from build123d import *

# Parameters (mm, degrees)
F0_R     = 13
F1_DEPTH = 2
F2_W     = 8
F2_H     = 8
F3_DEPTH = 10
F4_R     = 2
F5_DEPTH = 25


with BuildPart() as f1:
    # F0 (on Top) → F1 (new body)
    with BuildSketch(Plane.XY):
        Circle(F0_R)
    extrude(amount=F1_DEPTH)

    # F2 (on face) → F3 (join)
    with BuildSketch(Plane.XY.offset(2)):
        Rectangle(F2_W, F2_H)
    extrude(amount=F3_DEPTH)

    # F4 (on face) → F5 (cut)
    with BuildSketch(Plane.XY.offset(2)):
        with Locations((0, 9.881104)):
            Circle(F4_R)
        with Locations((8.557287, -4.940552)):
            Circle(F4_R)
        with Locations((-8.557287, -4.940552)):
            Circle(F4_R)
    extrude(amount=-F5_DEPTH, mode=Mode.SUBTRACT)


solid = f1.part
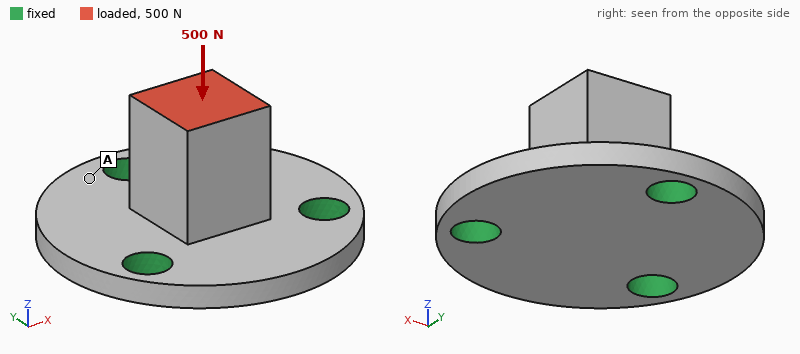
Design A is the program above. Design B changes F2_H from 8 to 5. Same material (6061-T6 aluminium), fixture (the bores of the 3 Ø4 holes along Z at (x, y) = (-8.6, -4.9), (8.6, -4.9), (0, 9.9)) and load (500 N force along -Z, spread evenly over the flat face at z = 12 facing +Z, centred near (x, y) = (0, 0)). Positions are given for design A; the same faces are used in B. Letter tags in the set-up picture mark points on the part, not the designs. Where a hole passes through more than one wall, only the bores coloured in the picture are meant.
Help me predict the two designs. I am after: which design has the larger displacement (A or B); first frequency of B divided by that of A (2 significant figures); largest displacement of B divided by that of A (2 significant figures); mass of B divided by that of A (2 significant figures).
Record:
B
0.91
1.5
0.85
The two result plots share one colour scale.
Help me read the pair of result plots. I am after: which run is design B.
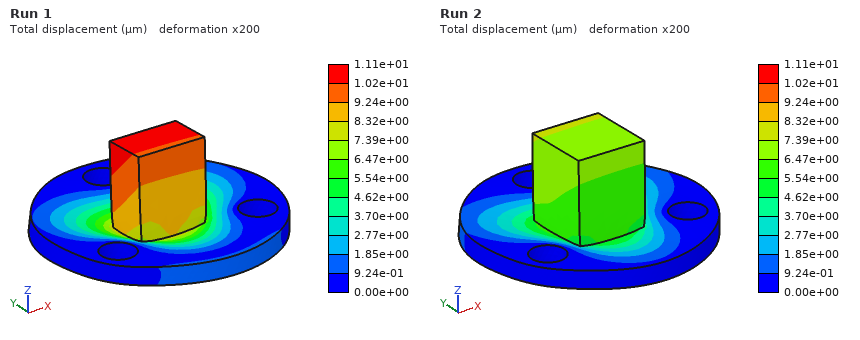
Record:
Run 1
